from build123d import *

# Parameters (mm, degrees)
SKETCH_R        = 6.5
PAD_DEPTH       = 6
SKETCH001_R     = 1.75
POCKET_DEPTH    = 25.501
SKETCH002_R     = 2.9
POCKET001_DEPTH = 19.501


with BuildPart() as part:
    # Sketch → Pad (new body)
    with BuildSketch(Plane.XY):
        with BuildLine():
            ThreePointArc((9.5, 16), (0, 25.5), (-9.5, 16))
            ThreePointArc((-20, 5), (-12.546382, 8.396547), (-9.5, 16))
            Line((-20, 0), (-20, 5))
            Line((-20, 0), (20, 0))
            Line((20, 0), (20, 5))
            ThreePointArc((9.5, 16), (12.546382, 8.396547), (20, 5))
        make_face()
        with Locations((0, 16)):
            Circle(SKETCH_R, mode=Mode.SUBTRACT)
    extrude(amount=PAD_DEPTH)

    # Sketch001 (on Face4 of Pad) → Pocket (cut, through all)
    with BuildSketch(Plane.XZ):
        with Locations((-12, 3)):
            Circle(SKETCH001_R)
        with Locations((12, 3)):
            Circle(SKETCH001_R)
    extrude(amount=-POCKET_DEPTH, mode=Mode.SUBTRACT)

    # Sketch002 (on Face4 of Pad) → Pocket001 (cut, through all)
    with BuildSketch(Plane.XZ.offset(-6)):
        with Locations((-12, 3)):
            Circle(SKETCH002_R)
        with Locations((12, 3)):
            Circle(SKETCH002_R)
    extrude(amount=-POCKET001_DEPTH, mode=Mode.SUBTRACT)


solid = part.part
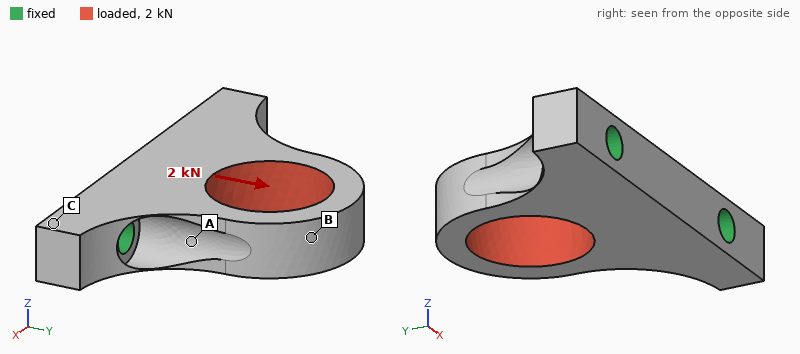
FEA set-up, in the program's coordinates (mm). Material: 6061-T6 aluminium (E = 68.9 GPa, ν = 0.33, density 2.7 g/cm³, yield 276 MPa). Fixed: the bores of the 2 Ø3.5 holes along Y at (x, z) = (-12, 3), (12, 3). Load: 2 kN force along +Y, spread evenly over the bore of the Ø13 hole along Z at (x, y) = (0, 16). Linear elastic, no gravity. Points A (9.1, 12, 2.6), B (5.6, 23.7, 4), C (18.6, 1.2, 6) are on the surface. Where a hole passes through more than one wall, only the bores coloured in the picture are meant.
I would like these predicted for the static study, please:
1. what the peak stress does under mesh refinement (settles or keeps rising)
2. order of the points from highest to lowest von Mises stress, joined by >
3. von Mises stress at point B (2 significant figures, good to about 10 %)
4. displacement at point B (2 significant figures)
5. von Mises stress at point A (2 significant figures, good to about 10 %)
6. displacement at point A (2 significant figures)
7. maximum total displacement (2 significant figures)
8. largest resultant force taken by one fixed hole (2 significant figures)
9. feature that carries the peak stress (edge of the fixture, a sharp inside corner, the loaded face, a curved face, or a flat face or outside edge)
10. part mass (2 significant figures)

keeps rising
A > B > C
18 MPa
13 µm
41 MPa
7.1 µm
19 µm
1.0 kN
edge of the fixture
6.8 g
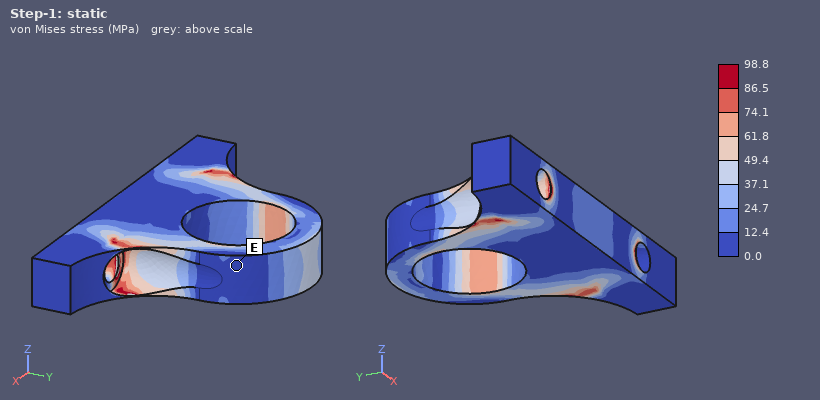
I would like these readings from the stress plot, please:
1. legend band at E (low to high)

0.0 to 12.4 MPa
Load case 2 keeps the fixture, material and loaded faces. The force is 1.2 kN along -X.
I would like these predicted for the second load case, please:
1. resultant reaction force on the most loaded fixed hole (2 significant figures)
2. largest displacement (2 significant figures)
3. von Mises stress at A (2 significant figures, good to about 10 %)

930 N
52 µm
72 MPa
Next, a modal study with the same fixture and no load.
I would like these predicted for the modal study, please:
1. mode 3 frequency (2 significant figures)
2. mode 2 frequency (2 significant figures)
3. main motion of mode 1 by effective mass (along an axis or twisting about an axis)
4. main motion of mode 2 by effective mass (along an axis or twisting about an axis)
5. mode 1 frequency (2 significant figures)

21 kHz
17 kHz
along Z
along X
9200 Hz
